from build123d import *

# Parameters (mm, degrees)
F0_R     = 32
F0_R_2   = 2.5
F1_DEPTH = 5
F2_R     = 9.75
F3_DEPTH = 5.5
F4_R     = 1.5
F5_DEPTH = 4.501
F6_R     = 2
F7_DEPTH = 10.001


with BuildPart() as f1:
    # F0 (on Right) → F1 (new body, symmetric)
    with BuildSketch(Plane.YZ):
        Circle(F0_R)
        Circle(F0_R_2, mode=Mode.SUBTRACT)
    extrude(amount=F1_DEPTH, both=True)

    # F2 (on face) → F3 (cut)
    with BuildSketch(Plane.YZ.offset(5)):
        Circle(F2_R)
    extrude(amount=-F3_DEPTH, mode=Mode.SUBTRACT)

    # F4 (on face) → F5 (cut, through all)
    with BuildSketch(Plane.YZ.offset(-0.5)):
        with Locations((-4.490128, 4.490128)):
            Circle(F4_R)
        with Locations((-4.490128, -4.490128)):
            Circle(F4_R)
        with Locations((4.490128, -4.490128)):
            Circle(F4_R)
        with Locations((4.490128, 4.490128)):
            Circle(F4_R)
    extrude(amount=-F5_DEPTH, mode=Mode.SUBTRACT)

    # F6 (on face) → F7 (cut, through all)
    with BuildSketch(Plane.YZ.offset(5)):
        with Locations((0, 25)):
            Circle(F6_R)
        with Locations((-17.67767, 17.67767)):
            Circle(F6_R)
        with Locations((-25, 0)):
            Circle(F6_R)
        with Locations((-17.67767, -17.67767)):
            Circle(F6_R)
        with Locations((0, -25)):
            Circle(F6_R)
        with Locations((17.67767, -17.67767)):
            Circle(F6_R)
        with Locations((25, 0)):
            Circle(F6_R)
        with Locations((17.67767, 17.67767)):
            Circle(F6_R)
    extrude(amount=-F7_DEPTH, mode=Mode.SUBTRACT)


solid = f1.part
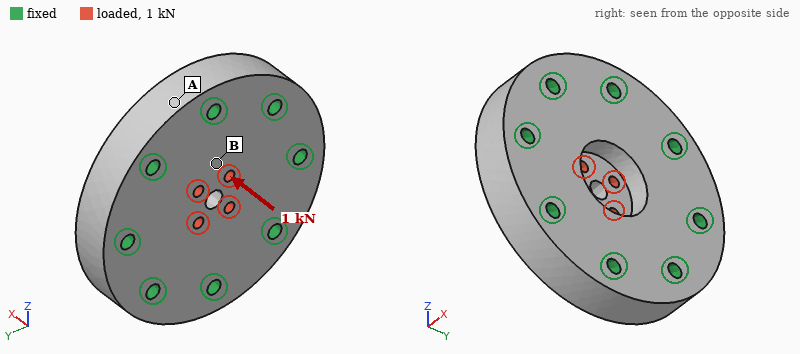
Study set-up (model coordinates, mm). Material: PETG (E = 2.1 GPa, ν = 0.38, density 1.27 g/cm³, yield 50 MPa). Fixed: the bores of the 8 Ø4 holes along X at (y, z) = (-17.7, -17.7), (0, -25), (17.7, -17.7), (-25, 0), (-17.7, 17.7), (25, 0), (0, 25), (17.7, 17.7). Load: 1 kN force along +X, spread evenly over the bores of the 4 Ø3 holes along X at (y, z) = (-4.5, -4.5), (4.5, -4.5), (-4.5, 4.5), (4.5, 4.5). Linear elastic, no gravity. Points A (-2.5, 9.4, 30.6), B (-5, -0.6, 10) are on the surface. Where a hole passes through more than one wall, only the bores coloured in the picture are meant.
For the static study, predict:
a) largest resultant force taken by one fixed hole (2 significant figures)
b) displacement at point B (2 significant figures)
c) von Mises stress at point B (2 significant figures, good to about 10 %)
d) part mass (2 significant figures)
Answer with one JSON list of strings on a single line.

["150 N", "0.085 mm", "8.0 MPa", "37 g"]
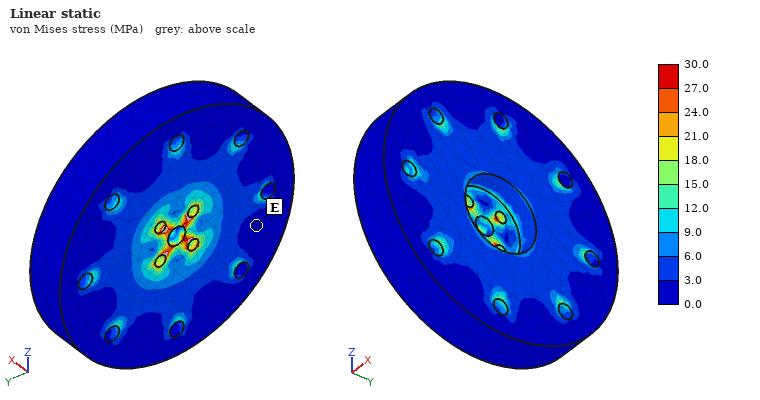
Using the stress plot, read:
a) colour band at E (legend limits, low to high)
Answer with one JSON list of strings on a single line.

["0.0 to 3.0 MPa"]
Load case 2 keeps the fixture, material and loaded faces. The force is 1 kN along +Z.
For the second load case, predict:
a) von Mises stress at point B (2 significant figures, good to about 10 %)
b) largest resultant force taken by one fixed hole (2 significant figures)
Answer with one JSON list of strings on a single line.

["3.2 MPa", "220 N"]
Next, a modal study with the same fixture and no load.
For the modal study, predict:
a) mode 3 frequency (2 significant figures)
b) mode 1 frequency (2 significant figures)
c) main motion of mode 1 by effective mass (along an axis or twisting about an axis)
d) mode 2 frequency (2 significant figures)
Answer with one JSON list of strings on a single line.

["11 kHz", "7400 Hz", "along X", "11 kHz"]
